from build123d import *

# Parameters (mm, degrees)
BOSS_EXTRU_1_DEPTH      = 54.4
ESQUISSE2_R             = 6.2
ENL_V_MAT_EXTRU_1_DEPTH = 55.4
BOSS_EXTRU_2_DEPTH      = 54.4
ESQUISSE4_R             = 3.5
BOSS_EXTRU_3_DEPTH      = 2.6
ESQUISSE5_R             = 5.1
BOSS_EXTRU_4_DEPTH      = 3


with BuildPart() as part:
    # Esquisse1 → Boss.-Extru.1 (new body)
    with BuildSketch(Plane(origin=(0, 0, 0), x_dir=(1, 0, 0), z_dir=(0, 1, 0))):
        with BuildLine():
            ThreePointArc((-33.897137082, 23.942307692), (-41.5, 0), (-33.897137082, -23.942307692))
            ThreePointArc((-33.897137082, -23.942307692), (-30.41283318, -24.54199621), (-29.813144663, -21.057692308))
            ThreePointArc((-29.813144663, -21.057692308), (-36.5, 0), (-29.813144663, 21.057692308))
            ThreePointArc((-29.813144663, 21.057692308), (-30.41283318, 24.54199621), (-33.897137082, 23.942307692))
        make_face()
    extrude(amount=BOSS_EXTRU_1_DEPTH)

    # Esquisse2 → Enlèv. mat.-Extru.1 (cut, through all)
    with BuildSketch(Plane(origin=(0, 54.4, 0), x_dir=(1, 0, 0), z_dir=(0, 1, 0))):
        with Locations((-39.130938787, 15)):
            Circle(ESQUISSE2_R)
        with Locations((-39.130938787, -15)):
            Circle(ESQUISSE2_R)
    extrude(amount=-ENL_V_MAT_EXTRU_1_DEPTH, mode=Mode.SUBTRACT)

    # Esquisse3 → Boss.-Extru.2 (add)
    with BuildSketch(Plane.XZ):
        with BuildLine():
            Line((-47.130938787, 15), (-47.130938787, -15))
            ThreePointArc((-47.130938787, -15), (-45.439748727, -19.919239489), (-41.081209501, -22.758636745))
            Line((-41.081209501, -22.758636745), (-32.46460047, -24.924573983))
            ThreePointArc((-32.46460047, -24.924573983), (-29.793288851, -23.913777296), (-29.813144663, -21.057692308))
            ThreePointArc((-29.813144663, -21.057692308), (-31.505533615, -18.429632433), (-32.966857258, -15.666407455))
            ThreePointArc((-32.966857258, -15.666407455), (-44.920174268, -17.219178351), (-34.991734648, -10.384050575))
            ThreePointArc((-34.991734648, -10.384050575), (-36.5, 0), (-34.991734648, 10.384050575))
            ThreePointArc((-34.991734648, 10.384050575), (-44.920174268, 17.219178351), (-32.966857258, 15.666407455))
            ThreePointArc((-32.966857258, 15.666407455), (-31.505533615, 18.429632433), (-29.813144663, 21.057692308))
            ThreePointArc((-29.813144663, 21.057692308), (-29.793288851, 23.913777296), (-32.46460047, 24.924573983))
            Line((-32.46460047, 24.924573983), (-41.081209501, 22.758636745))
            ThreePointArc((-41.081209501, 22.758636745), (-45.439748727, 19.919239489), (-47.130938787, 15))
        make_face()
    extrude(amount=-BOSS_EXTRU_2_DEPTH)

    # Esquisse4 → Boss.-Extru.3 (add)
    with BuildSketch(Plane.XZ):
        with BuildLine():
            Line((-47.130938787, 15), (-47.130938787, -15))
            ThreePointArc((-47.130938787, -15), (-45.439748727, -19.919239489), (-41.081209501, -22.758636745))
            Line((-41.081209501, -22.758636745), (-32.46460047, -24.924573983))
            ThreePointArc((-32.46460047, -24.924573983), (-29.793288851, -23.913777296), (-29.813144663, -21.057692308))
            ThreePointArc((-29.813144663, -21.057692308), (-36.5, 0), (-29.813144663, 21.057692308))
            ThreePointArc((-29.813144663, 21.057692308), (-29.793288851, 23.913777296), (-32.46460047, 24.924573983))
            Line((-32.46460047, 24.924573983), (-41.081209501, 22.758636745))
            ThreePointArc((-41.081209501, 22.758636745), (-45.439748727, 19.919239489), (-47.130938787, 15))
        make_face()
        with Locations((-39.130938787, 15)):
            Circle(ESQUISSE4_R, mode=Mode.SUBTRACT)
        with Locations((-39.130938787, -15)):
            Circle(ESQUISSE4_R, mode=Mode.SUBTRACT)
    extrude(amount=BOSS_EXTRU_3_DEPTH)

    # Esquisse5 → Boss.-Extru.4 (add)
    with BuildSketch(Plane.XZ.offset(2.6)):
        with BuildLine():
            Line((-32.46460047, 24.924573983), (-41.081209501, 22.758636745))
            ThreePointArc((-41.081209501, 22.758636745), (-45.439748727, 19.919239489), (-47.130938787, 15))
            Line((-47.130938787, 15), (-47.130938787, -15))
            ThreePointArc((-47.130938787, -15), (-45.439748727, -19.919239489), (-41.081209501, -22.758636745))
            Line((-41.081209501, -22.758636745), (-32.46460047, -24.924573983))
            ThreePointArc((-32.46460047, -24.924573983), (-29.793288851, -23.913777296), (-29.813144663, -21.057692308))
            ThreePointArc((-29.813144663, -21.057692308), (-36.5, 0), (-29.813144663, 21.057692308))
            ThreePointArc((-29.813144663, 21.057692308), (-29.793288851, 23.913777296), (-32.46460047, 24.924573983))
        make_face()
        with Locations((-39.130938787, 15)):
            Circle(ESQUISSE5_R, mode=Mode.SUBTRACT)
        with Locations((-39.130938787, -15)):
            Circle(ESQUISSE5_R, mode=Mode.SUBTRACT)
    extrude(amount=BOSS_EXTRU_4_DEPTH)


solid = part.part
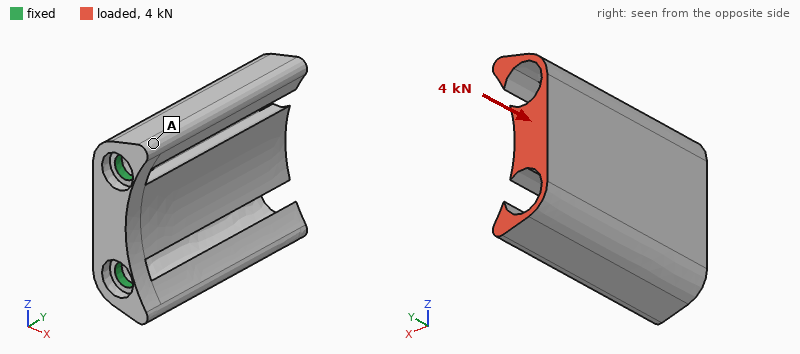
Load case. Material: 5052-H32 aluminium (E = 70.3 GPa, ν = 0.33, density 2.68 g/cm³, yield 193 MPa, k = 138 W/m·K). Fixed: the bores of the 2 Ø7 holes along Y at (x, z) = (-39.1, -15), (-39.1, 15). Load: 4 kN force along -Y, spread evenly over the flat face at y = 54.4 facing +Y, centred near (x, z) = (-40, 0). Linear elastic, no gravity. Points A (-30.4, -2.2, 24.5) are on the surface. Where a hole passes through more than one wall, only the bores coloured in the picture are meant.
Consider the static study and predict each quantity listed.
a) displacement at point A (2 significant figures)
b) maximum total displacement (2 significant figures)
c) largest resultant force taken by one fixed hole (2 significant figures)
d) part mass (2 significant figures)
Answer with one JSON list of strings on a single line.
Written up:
["9.0 µm", "18 µm", "2.0 kN", "61 g"]
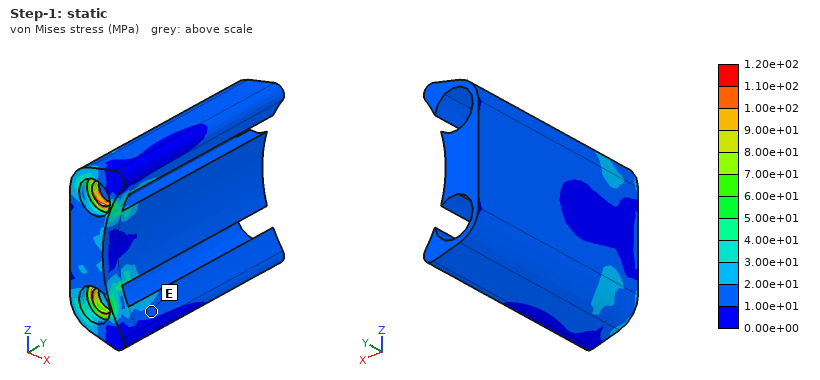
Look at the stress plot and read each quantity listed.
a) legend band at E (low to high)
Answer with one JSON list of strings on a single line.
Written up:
["1.00e+01 to 2.00e+01 MPa"]
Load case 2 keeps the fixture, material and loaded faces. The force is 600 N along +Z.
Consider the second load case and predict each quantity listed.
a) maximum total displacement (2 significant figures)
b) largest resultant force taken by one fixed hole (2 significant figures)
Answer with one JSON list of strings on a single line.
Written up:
["0.14 mm", "1.1 kN"]
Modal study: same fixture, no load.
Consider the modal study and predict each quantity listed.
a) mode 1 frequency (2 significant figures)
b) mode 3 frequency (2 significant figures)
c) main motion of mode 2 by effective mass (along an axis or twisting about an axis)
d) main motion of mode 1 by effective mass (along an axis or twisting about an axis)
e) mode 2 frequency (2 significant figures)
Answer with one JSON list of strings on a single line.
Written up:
["1600 Hz", "4000 Hz", "along Z", "along X", "3200 Hz"]
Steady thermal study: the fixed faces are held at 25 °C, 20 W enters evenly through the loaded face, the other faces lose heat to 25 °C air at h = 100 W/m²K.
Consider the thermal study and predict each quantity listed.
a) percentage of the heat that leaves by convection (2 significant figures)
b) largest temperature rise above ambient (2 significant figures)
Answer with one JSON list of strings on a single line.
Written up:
["46 %", "18 K"]
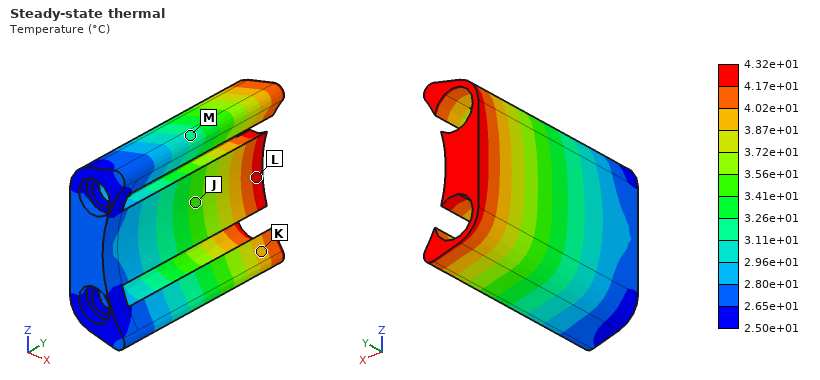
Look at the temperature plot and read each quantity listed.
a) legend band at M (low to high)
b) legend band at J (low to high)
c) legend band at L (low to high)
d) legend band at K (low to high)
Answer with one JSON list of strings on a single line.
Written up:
["3.11e+01 to 3.26e+01 °C", "3.41e+01 to 3.56e+01 °C", "4.17e+01 to 4.32e+01 °C", "3.87e+01 to 4.02e+01 °C"]
